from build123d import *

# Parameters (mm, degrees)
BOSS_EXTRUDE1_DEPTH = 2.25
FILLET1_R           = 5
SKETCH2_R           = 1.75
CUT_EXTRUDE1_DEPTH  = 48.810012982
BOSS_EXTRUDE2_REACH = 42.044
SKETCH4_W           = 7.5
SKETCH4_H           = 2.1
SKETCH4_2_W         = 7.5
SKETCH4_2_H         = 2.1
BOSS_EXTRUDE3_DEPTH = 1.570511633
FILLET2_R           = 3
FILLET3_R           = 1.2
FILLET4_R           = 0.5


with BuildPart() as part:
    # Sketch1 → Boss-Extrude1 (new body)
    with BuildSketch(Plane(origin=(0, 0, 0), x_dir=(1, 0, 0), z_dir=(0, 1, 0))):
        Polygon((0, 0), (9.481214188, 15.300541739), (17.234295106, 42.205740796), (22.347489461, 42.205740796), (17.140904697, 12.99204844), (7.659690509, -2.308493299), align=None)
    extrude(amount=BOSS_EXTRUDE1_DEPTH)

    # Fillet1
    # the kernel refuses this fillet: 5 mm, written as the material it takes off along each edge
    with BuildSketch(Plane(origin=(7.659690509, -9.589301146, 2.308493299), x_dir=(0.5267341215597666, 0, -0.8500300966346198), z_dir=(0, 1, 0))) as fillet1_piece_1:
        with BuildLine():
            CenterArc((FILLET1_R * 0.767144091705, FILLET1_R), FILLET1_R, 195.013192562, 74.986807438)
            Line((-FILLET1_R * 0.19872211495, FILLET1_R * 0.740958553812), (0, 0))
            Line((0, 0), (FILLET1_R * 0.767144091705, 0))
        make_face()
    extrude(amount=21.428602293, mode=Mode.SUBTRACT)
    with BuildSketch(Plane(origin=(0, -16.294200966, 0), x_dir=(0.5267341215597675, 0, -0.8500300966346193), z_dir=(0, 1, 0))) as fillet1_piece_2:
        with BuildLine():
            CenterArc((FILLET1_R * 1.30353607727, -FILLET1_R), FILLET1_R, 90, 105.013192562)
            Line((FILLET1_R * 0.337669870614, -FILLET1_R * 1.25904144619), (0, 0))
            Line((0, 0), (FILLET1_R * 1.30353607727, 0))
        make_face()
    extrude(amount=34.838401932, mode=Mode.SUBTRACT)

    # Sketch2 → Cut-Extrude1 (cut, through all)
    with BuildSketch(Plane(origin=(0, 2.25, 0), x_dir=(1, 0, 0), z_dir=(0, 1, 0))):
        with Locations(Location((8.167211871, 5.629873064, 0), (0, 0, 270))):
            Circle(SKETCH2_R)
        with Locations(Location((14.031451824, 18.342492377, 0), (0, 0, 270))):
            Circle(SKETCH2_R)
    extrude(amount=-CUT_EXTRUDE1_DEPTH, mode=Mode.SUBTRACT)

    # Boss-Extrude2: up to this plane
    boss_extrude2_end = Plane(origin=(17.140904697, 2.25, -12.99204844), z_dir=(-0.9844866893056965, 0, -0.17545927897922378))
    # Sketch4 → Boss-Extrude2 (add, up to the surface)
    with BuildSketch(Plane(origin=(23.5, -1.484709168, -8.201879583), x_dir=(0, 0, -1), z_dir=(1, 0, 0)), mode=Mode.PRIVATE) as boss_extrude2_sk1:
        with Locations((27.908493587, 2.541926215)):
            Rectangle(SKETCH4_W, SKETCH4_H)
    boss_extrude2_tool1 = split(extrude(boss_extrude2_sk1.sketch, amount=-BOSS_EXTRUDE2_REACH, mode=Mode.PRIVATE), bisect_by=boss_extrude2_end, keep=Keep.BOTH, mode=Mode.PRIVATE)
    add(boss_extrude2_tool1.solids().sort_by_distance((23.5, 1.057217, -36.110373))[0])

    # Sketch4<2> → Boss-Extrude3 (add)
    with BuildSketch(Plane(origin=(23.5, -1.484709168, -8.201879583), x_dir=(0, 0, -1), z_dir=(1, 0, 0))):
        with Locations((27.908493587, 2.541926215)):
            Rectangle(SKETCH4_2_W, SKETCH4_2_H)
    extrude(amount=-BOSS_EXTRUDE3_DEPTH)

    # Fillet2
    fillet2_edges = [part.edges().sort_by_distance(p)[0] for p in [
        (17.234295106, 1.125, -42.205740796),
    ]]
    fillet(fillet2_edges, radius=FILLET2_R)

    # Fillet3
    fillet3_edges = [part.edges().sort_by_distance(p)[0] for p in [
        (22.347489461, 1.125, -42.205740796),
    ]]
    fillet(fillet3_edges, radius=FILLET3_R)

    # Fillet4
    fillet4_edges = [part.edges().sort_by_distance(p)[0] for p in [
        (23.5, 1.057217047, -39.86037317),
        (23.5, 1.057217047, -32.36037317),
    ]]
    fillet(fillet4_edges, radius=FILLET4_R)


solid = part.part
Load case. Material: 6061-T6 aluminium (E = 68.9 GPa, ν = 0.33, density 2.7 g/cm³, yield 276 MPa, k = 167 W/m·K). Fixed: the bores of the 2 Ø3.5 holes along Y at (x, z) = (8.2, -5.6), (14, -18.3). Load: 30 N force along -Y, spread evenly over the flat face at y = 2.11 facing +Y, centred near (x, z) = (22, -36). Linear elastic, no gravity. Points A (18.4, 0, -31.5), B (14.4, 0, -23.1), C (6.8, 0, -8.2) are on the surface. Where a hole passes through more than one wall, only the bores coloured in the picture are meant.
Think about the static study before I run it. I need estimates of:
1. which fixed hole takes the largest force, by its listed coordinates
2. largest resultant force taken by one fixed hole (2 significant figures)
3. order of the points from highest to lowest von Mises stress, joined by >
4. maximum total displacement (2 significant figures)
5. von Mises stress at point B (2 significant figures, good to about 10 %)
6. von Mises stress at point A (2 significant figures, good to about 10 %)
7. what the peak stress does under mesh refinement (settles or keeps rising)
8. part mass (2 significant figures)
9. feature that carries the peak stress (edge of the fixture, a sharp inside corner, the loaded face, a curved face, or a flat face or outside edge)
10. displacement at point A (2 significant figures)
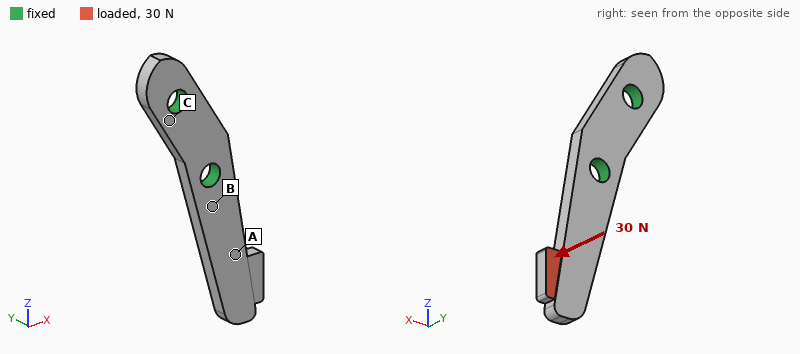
(14, -18.3)
30 N
B > A > C
0.19 mm
71 MPa
38 MPa
keeps rising
1.9 g
edge of the fixture
0.074 mm
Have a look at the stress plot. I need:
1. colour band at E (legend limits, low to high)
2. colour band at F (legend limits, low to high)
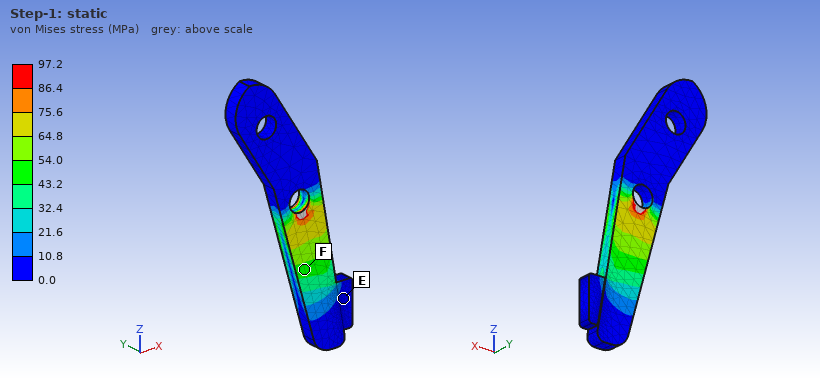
0.0 to 10.8 MPa
43.2 to 54.0 MPa
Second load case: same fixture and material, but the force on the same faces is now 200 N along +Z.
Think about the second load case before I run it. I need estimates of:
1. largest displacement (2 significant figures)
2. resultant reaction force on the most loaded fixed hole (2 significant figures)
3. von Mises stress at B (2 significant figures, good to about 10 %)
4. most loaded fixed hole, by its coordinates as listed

0.15 mm
200 N
38 MPa
(14, -18.3)
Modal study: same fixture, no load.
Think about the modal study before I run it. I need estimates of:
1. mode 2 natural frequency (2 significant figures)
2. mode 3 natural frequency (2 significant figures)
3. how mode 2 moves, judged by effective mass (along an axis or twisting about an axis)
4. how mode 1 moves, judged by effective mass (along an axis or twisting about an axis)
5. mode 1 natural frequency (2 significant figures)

9000 Hz
18 kHz
along X
along Y
3500 Hz
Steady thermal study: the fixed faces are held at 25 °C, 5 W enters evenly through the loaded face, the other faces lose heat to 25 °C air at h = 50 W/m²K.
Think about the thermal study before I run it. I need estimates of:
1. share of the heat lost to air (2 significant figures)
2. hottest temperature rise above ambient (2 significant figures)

8.7 %
37 K
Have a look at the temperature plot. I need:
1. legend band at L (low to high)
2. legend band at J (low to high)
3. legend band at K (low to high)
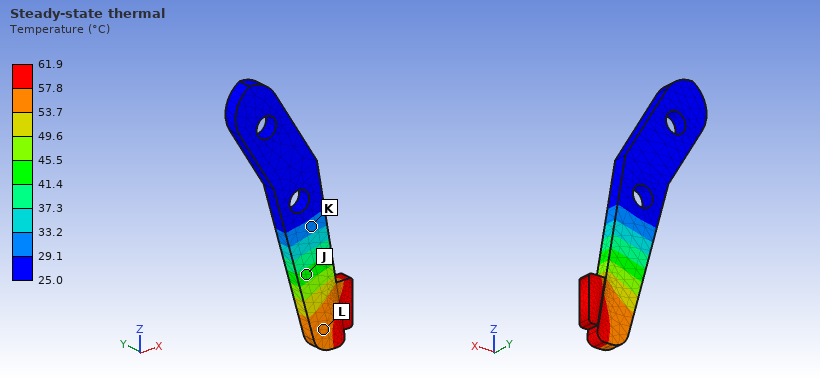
53.7 to 57.8 °C
41.4 to 45.5 °C
29.1 to 33.2 °C
